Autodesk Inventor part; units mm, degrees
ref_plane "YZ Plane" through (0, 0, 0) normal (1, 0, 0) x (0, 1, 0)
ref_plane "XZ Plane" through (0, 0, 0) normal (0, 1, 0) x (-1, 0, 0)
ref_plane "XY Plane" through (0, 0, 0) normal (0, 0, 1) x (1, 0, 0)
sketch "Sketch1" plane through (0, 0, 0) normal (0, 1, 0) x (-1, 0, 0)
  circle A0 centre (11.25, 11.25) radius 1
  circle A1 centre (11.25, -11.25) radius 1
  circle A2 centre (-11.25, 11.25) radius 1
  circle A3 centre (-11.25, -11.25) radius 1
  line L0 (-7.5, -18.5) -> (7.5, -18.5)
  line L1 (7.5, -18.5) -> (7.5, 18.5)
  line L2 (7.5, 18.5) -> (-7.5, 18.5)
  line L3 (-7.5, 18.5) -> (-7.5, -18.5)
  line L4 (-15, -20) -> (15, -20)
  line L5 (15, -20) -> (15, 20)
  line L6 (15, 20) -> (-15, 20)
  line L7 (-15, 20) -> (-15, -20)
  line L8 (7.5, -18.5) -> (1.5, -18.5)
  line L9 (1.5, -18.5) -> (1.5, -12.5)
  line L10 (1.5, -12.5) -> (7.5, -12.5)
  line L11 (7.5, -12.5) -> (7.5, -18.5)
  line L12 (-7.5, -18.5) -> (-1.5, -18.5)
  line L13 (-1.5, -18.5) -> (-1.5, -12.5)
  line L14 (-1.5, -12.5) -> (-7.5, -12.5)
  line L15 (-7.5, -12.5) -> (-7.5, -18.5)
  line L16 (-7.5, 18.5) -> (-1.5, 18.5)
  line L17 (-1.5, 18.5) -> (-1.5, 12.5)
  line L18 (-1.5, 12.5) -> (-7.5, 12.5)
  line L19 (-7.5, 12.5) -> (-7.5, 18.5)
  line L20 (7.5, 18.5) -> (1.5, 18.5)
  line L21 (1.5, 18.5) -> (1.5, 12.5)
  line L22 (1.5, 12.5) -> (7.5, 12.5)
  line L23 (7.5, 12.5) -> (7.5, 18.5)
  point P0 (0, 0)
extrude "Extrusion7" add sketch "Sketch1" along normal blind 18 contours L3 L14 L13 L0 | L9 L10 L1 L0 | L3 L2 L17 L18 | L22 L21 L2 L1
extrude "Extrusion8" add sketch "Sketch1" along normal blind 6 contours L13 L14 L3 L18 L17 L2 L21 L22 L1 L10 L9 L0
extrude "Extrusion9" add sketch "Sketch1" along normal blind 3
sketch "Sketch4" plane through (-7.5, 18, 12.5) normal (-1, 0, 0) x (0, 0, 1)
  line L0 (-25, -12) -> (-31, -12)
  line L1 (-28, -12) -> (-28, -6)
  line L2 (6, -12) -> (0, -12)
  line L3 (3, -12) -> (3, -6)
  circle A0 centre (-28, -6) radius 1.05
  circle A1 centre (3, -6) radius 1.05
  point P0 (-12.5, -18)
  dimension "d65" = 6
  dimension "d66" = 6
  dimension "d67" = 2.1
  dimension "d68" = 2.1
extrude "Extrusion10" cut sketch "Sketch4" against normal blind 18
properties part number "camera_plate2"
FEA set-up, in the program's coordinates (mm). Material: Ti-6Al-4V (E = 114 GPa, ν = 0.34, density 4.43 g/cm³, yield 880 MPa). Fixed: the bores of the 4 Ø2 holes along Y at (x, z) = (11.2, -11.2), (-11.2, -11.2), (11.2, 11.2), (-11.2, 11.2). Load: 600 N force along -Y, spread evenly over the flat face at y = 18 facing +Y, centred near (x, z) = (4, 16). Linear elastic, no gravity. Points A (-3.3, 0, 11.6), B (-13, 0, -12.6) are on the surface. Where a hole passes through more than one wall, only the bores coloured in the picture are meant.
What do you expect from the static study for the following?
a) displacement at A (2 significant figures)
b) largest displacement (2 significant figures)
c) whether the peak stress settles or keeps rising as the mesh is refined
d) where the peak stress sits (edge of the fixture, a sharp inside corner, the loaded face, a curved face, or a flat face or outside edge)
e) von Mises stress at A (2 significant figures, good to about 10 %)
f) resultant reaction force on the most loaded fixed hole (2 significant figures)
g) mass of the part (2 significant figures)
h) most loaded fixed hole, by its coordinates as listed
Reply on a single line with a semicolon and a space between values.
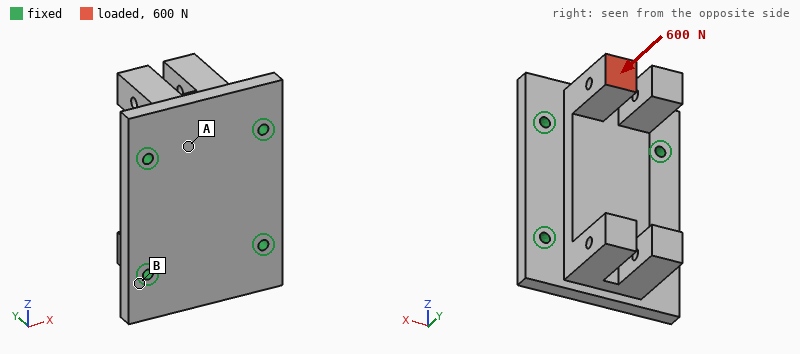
3.7 µm; 17 µm; keeps rising; edge of the fixture; 15 MPa; 500 N; 30 g; (11.2, 11.2)
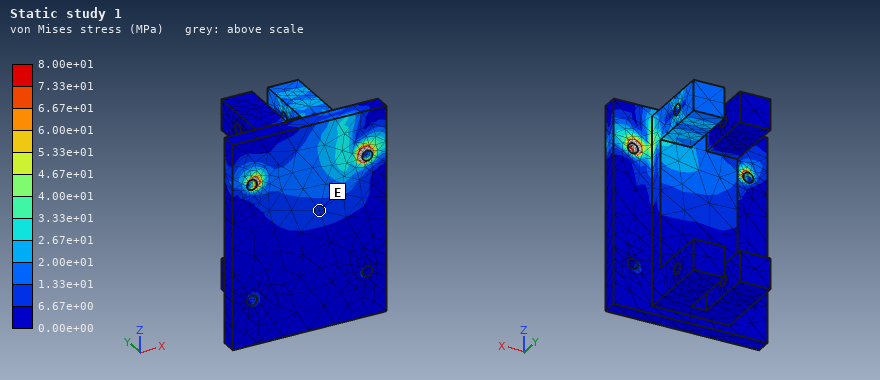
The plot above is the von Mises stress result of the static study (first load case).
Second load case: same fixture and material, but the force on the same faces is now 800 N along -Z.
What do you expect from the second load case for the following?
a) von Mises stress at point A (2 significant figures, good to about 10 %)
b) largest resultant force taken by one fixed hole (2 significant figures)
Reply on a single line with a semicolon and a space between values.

63 MPa; 470 N
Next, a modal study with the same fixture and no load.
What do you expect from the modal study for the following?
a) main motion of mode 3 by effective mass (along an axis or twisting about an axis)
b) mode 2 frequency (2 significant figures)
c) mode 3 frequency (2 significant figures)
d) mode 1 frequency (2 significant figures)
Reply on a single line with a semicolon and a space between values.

along X; 12 kHz; 17 kHz; 12 kHz
